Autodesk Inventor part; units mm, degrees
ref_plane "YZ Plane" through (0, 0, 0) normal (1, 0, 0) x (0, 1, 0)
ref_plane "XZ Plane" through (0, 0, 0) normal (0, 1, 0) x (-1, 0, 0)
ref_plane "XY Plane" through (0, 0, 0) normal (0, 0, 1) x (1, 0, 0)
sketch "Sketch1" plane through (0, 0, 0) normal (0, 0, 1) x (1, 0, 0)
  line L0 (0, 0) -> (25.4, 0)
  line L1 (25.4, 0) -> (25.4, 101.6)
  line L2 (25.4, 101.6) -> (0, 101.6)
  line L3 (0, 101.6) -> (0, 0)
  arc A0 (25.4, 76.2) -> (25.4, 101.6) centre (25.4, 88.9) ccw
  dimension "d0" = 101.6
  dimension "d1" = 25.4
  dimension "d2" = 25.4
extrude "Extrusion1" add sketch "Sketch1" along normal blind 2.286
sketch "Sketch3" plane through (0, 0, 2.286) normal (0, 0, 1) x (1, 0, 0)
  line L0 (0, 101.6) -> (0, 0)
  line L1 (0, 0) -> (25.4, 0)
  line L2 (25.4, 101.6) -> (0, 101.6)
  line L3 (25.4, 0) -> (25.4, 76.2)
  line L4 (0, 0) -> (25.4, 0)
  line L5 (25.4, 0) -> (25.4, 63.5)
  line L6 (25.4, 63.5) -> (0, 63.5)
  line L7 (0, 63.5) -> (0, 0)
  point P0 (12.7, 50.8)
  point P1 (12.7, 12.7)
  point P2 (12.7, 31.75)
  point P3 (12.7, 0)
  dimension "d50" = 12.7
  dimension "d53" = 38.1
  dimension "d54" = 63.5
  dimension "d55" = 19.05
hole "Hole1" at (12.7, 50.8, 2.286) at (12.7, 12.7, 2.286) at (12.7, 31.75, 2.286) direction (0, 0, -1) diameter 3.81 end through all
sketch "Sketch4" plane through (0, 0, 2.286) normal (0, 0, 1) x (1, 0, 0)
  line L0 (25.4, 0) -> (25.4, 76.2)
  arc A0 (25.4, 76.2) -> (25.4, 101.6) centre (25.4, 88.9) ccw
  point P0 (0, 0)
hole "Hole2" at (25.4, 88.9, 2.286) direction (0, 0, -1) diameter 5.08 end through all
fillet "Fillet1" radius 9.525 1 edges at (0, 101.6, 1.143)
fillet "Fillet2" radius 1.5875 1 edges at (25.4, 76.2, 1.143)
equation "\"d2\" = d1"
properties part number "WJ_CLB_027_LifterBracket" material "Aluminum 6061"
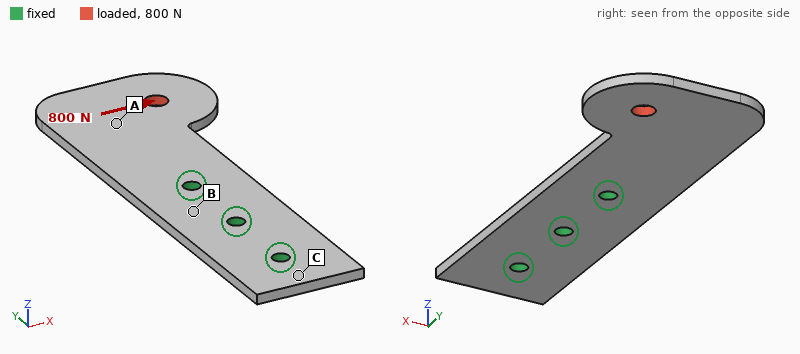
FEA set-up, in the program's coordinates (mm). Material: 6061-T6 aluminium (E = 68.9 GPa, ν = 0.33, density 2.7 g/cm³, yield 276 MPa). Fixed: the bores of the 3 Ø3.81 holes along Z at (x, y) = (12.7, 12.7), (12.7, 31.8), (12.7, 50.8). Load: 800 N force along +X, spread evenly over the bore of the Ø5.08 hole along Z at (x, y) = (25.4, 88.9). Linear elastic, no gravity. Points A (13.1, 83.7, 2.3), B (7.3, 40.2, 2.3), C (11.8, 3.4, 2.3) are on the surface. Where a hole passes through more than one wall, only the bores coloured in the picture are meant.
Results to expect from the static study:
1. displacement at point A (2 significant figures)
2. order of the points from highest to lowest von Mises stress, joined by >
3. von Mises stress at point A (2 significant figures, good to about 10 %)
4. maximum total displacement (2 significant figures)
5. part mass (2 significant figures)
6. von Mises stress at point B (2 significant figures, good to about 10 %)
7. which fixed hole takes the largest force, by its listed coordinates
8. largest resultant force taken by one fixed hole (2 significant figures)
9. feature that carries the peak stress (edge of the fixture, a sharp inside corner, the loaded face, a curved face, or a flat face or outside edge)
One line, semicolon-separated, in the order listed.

0.13 mm; B > A > C; 29 MPa; 0.23 mm; 17 g; 46 MPa; (12.7, 50.8); 1.8 kN; edge of the fixture
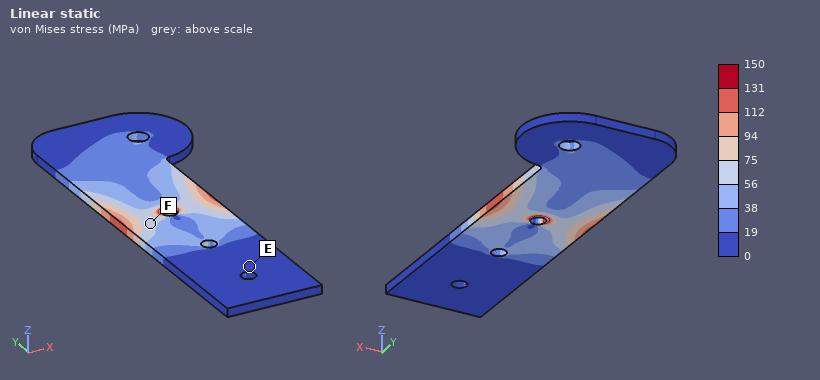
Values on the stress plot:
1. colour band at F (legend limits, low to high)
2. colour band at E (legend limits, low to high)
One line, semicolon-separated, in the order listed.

56 to 75 MPa; 0 to 19 MPa
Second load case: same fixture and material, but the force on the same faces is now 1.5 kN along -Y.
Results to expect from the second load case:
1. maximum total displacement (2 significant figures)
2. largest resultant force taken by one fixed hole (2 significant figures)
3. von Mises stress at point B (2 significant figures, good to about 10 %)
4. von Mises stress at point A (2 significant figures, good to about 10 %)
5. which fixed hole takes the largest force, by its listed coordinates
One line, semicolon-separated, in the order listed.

0.18 mm; 1.3 kN; 21 MPa; 21 MPa; (12.7, 50.8)
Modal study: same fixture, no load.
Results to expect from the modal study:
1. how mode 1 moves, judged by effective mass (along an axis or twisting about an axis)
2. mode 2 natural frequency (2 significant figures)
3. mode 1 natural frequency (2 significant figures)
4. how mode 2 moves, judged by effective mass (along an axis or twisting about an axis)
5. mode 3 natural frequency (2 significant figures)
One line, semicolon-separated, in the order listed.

along Z; 1800 Hz; 640 Hz; twisting about Y; 4200 Hz
